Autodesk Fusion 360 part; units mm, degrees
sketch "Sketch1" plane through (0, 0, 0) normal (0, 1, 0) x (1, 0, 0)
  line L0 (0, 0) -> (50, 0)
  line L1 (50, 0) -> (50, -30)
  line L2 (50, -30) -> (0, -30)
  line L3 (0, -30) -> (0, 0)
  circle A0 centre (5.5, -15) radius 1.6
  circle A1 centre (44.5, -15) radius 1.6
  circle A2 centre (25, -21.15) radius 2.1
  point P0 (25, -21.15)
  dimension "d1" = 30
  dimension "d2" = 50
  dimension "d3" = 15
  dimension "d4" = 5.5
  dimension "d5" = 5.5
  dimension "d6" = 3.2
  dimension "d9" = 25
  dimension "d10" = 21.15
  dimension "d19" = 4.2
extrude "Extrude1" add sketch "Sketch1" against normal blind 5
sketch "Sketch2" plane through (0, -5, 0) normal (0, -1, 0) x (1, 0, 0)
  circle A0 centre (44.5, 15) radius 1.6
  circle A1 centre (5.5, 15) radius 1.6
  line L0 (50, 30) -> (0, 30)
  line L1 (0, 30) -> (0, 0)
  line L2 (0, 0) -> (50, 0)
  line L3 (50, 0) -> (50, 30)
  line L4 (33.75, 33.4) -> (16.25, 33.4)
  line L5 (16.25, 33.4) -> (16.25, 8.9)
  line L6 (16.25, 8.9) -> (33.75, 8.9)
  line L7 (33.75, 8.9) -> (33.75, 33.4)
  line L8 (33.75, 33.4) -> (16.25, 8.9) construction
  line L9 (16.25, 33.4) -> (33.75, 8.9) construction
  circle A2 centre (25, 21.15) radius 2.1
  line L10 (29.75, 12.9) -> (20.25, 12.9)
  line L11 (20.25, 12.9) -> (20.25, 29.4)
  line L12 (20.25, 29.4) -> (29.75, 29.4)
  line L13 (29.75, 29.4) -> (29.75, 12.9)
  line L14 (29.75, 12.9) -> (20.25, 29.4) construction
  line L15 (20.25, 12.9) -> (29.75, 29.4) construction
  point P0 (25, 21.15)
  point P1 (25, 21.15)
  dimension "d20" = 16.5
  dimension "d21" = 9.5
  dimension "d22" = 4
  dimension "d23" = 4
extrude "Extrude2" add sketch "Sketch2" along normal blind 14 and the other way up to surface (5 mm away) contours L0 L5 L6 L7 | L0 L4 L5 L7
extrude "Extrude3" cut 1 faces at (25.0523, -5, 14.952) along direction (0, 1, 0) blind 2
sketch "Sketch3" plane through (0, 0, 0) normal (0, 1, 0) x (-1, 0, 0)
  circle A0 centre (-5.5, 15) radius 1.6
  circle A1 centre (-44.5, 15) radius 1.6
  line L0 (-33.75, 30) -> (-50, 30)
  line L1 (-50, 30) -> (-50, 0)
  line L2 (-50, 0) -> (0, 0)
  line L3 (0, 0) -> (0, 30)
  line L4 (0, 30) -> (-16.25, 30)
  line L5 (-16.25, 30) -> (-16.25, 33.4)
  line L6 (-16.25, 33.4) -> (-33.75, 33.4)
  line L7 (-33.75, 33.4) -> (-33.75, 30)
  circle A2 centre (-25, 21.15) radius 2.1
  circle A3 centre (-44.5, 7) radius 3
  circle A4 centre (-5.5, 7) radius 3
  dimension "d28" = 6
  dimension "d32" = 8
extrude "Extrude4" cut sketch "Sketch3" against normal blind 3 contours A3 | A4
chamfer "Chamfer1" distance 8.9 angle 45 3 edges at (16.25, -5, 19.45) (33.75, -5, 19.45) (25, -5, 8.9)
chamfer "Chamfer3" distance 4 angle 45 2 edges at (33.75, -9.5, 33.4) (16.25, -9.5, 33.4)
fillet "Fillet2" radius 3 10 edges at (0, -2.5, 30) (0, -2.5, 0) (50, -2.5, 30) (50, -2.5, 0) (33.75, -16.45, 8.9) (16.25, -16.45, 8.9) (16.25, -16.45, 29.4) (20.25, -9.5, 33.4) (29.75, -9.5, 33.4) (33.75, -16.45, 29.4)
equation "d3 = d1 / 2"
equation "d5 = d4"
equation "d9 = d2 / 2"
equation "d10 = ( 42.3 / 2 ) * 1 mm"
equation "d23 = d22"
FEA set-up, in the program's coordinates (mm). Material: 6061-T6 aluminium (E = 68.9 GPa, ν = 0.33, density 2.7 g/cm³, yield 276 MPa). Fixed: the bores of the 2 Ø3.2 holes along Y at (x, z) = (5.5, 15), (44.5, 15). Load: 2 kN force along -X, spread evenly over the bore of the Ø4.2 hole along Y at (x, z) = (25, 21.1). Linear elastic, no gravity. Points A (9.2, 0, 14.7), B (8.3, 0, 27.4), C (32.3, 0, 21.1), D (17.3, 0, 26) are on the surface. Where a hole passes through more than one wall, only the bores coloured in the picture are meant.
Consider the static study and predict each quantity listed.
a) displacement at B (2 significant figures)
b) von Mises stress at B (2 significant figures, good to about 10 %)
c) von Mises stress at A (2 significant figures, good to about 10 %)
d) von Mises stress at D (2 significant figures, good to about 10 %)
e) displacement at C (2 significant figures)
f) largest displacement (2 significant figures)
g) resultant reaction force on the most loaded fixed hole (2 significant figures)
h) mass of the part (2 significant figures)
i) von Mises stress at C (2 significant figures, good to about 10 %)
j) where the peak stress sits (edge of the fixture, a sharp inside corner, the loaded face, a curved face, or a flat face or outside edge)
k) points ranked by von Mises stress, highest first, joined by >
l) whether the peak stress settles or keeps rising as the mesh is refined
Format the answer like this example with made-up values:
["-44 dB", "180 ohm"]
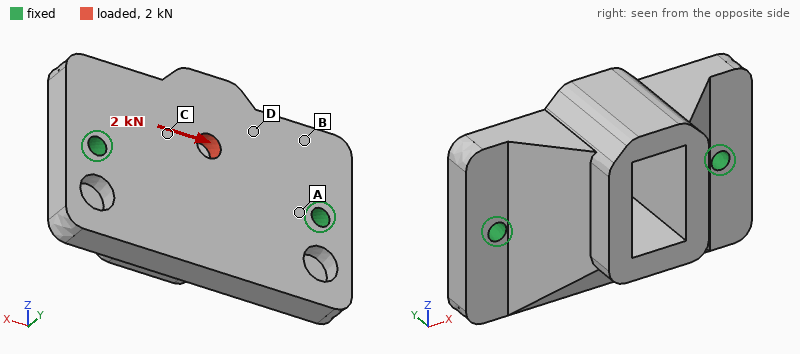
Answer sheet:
["4.2 µm", "5.6 MPa", "21 MPa", "12 MPa", "4.4 µm", "7.7 µm", "1.0 kN", "36 g", "29 MPa", "edge of the fixture", "C > A > D > B", "keeps rising"]
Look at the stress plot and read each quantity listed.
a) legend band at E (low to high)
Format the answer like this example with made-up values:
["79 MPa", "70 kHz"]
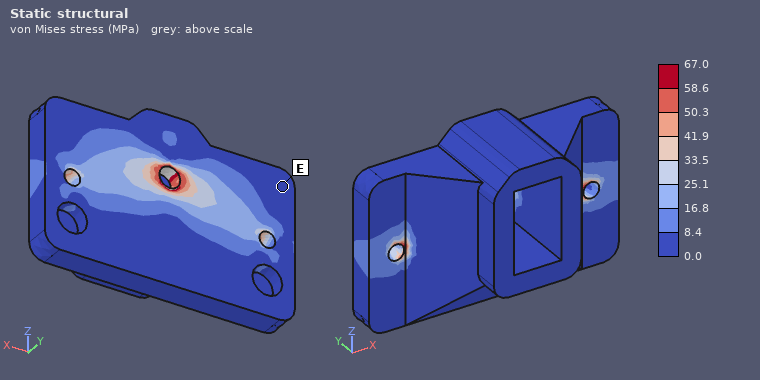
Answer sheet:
["0.0 to 8.4 MPa"]
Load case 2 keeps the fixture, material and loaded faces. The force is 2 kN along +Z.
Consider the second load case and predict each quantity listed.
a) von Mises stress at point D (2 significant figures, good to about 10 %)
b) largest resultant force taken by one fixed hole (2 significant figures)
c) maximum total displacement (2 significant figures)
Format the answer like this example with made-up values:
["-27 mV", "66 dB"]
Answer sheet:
["14 MPa", "1.0 kN", "11 µm"]
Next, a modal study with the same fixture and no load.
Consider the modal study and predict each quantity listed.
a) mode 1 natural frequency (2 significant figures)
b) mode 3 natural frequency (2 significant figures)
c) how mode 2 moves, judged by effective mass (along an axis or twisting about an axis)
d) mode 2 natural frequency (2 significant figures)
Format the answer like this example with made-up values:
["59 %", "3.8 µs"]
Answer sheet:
["6300 Hz", "22 kHz", "along Y", "14 kHz"]
